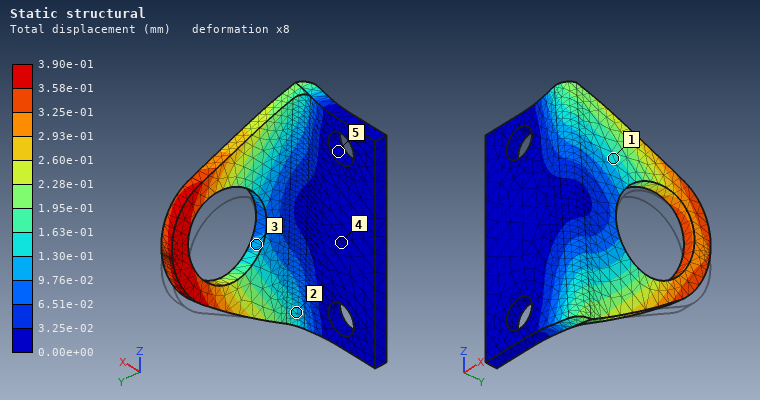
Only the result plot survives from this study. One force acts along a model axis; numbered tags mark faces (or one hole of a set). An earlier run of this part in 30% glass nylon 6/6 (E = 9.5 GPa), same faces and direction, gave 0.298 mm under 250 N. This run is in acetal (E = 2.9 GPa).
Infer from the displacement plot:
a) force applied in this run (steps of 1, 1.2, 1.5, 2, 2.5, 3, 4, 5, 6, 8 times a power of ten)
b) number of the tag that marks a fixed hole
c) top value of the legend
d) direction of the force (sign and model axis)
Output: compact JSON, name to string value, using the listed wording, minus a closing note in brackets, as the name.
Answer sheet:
{"force applied in this run": "100 N", "number of the tag that marks a fixed hole": "5", "top value of the legend": "3.90e-01 mm", "direction of the force": "+Z"}
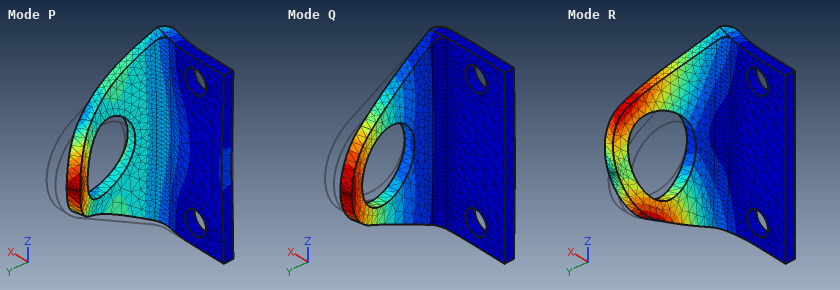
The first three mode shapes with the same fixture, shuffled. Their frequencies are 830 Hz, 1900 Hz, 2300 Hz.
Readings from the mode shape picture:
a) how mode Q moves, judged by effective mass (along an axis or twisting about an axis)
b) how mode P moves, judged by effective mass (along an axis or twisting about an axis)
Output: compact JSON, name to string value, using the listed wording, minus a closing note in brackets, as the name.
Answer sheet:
{"how mode Q moves, judged by effective mass": "along X", "how mode P moves, judged by effective mass": "along Y"}
